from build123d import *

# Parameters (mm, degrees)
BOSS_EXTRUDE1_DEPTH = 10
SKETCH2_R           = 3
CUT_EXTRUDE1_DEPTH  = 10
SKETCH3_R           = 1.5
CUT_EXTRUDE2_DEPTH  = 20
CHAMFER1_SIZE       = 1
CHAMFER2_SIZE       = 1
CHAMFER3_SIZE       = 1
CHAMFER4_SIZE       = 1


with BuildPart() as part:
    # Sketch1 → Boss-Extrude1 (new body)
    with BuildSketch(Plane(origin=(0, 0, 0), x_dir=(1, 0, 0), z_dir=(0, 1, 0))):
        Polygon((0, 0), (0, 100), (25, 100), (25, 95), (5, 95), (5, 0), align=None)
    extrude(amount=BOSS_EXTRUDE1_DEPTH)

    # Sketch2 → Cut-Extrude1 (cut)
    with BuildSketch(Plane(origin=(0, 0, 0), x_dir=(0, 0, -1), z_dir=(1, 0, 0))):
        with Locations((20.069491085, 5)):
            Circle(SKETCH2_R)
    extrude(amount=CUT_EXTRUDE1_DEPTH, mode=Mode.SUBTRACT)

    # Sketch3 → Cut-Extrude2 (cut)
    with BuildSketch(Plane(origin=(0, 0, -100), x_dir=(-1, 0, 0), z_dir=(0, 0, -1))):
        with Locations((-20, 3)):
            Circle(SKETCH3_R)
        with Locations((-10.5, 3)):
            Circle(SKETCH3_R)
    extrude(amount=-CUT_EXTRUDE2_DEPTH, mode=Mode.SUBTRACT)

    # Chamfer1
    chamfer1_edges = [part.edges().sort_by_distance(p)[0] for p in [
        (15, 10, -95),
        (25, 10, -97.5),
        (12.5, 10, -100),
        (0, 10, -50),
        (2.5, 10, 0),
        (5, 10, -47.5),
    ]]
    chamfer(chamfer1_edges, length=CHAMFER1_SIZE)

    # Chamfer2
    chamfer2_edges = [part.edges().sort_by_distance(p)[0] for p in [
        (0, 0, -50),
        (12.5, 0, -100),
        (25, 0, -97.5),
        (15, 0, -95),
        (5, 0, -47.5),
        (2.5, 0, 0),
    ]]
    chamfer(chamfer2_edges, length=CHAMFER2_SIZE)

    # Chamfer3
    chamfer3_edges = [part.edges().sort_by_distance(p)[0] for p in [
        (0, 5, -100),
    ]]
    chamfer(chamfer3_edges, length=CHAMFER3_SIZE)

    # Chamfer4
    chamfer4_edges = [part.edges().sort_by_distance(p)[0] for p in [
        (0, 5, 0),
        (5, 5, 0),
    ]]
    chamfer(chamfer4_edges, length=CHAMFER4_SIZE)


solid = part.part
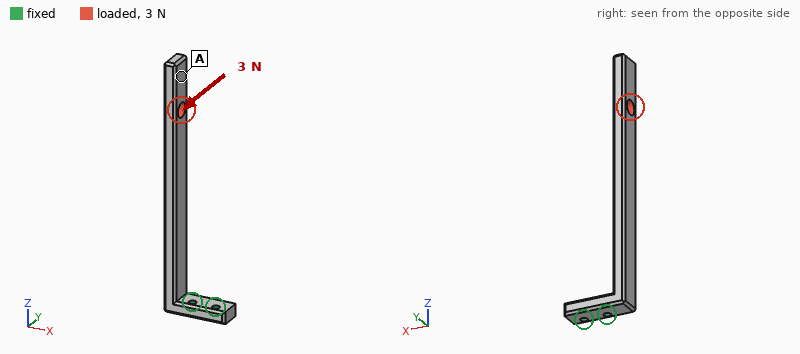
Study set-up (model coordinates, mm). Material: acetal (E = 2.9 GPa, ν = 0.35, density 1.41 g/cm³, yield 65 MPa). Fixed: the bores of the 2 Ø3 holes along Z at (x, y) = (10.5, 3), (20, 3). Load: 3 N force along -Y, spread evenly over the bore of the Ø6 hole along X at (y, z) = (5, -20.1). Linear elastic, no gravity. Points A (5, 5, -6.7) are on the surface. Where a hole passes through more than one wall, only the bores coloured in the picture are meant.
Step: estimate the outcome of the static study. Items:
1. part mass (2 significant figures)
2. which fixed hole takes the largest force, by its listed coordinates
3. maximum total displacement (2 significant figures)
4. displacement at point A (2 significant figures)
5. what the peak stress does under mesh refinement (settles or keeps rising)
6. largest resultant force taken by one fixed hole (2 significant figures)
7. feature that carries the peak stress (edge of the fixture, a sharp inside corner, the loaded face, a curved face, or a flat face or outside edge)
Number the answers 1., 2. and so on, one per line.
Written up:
1. 7.8 g
2. (10.5, 3)
3. 1.1 mm
4. 0.97 mm
5. keeps rising
6. 4.5 N
7. edge of the fixture
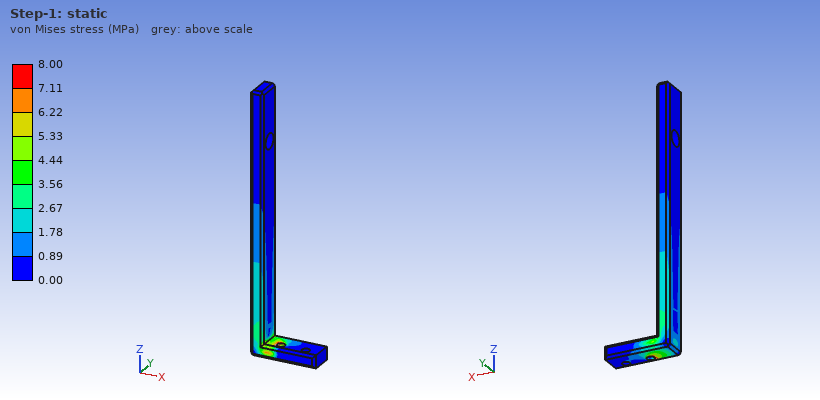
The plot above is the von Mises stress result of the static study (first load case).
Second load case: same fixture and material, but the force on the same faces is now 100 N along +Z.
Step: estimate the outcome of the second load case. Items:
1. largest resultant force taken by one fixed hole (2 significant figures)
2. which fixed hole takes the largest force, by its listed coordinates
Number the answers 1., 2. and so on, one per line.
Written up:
1. 110 N
2. (10.5, 3)
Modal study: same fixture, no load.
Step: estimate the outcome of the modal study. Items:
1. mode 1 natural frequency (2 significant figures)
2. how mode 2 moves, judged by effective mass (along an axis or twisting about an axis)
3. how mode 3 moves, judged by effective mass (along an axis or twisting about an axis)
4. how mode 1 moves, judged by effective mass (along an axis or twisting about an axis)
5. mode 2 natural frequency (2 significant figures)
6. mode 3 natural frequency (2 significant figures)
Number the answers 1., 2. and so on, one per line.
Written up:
1. 110 Hz
2. along Y
3. along X
4. along X
5. 180 Hz
6. 660 Hz
